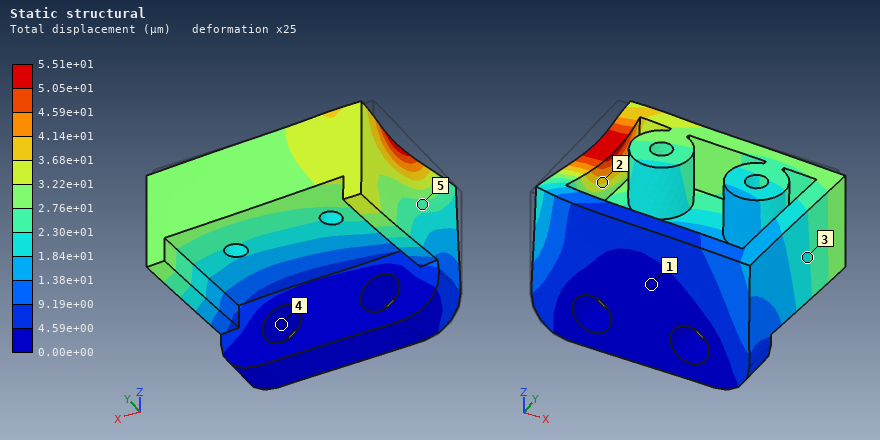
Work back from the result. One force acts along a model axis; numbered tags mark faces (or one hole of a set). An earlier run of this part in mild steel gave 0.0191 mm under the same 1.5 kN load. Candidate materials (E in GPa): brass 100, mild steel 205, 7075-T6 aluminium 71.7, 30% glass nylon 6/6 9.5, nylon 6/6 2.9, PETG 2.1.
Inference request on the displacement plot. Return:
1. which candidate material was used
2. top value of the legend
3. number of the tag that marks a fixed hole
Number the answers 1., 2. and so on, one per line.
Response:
1. 7075-T6 aluminium
2. 5.51e+01 µm
3. 4
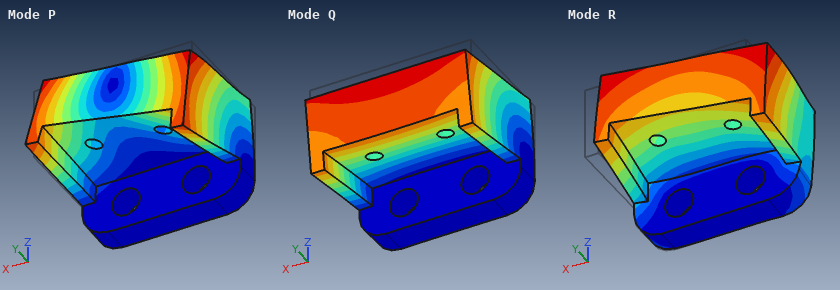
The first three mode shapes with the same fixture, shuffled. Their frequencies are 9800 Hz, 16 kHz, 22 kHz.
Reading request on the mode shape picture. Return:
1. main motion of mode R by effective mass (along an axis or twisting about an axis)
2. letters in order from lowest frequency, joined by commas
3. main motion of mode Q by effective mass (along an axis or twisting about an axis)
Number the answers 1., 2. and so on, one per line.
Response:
1. along X
2. Q, P, R
3. along Z
